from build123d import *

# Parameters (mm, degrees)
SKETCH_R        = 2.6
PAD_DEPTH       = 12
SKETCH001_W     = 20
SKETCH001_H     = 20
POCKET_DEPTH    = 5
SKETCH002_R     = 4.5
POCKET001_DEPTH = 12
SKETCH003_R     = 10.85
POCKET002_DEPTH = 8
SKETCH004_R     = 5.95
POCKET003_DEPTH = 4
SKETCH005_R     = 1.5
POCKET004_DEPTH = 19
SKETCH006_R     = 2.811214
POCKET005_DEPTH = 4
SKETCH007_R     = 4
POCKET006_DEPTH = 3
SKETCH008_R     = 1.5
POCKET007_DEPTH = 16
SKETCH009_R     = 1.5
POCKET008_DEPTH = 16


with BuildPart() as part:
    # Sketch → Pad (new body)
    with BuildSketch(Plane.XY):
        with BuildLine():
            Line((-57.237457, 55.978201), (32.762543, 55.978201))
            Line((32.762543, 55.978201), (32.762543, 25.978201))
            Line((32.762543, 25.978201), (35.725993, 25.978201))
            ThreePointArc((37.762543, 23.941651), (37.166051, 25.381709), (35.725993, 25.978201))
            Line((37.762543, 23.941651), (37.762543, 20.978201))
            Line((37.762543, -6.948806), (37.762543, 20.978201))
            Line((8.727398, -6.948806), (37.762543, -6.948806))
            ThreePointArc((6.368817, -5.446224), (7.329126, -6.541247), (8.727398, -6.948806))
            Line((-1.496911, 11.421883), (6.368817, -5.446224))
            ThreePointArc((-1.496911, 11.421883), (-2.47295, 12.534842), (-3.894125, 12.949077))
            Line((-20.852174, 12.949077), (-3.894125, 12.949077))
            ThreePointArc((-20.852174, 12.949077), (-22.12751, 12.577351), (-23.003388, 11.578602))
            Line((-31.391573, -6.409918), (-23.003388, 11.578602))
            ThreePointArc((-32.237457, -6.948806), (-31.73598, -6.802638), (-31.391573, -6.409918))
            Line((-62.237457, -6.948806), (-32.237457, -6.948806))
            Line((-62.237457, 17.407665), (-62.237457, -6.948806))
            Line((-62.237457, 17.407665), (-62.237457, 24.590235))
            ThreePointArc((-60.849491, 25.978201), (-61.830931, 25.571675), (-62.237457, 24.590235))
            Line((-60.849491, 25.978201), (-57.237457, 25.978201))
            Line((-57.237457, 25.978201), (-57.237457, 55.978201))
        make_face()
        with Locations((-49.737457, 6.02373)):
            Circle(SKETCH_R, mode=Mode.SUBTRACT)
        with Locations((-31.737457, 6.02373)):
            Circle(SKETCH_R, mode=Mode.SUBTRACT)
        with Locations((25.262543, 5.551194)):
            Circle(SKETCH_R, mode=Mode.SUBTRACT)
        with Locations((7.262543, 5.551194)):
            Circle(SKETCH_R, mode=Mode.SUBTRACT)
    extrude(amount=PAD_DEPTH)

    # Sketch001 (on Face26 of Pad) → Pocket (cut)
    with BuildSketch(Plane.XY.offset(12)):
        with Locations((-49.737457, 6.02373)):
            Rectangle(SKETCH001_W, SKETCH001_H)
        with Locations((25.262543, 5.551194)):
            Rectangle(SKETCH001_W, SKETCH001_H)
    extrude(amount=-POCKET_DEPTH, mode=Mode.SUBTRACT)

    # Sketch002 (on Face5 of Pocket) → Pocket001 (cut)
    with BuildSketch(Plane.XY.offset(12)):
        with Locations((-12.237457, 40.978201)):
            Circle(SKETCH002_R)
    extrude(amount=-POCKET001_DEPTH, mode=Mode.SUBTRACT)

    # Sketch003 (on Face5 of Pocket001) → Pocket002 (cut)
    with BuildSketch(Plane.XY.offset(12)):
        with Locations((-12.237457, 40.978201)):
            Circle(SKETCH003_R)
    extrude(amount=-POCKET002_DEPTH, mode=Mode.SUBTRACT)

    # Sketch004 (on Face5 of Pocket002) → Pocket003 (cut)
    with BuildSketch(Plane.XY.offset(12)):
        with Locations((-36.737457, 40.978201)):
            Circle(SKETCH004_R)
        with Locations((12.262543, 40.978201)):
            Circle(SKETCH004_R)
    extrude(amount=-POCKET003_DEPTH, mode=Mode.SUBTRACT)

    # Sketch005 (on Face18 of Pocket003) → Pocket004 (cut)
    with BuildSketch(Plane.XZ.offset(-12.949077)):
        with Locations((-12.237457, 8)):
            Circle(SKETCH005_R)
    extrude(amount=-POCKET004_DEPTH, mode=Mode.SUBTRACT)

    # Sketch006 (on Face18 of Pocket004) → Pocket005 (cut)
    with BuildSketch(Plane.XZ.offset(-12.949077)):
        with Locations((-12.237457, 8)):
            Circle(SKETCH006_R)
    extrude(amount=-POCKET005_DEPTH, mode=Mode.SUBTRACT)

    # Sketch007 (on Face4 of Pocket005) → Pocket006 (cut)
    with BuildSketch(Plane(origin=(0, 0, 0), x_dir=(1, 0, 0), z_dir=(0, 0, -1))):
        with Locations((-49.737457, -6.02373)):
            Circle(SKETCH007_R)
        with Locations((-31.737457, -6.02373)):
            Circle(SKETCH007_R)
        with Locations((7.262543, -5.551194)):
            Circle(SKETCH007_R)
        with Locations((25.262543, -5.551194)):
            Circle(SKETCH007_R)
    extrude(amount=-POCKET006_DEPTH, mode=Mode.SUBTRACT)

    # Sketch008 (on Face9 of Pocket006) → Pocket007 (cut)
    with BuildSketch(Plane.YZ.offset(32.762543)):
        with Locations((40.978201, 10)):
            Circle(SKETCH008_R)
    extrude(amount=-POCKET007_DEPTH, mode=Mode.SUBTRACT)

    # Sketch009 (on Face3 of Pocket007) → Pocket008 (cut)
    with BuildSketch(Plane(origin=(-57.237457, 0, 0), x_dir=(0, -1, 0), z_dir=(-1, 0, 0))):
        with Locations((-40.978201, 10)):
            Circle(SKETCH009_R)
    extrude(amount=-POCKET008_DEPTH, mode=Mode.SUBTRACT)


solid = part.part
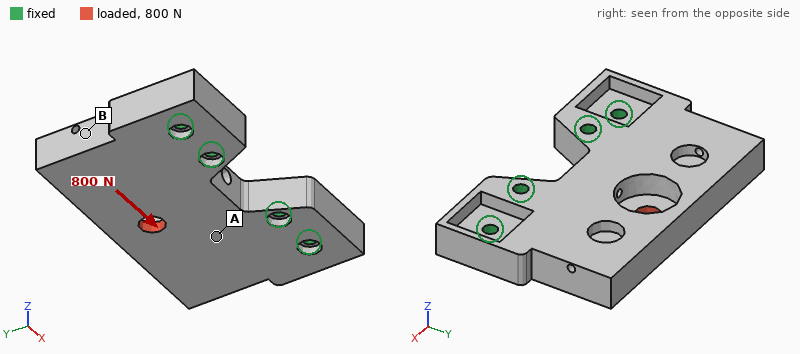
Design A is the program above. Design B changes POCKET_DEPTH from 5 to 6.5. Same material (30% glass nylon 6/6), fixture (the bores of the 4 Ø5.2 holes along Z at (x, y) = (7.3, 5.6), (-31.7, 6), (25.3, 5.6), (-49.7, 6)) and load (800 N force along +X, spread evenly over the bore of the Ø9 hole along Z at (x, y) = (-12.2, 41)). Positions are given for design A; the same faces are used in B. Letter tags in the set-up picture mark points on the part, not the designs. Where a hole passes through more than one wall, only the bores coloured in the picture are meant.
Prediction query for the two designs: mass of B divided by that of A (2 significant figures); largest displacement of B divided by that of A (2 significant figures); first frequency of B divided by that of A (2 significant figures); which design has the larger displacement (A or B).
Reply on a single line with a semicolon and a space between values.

0.98; 1.1; 0.97; B
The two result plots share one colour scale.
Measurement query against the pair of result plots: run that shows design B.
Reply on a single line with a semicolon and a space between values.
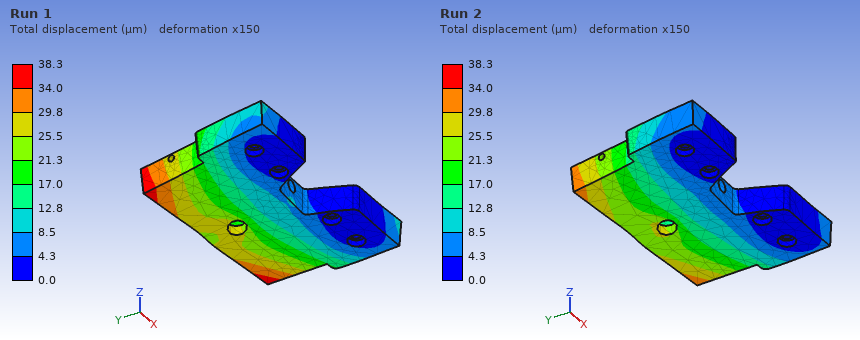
Run 1
